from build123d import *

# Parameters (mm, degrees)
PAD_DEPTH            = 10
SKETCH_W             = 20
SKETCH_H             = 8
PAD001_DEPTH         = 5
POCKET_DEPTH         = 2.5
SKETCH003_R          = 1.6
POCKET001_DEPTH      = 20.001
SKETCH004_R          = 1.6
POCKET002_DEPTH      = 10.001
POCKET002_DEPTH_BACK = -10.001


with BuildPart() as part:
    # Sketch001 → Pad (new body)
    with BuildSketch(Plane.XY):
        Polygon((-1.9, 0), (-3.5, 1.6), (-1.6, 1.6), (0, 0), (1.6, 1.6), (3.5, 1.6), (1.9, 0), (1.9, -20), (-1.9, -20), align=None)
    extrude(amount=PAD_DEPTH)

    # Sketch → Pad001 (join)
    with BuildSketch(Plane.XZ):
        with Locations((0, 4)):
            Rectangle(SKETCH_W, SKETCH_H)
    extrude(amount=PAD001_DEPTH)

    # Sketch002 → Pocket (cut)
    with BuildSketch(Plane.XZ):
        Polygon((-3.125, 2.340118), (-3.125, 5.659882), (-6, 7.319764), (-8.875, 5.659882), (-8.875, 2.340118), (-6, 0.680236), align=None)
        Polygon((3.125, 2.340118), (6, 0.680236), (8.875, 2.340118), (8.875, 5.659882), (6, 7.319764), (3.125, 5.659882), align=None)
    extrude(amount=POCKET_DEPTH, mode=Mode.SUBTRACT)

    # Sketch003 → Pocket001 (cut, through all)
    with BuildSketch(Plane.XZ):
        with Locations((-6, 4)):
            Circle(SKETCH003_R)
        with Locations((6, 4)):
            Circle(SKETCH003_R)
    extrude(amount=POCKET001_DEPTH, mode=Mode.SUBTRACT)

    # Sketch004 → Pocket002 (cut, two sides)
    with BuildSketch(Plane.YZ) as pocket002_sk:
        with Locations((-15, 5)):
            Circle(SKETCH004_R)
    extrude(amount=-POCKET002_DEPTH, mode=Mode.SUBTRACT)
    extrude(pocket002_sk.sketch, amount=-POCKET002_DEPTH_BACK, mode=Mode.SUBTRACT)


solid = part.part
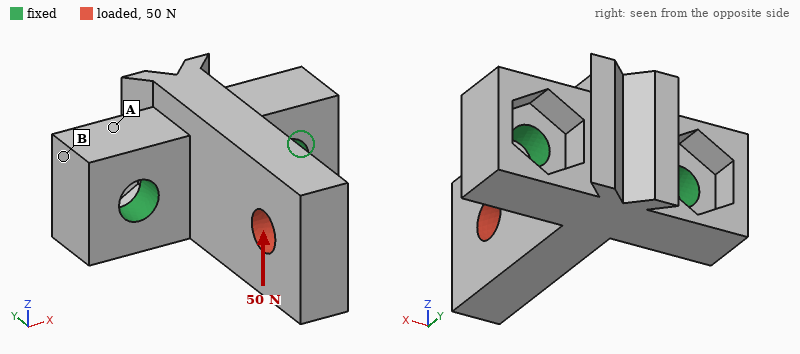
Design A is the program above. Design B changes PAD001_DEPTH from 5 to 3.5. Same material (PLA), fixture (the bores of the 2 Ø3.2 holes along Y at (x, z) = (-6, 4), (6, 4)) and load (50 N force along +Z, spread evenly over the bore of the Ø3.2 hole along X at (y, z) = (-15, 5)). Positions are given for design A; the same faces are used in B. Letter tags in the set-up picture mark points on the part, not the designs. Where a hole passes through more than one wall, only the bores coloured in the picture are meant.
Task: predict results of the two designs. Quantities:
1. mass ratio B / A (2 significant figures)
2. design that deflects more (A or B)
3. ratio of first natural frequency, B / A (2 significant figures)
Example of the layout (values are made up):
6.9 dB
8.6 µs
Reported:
0.86
B
0.60
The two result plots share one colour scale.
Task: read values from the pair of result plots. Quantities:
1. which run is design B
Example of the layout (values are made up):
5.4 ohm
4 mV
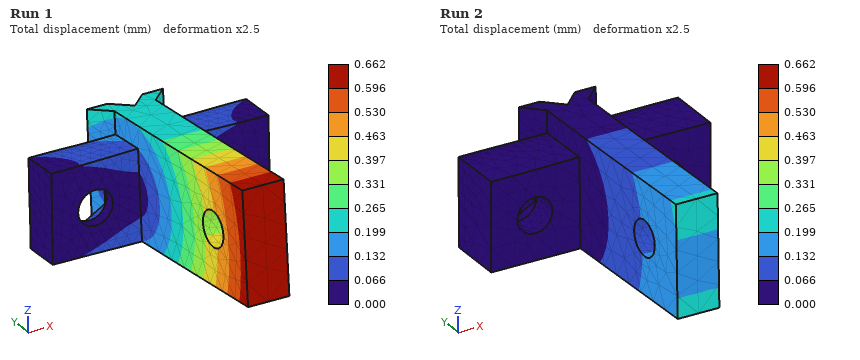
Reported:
Run 1
